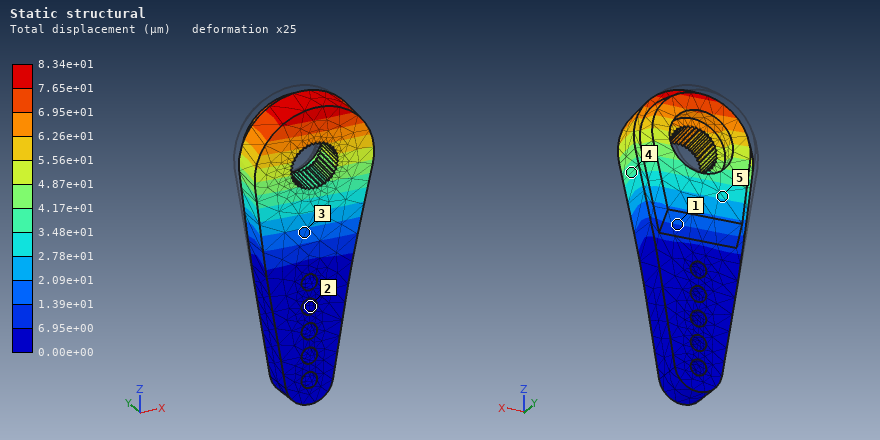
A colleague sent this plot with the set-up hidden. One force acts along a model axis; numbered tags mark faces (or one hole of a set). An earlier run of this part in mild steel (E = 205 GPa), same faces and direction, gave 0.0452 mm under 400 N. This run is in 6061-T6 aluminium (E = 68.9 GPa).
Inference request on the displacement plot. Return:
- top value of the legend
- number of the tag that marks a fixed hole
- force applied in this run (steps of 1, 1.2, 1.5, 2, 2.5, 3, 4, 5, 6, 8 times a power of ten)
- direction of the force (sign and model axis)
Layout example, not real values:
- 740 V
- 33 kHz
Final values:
- 8.34e+01 µm
- 2
- 250 N
- -Y
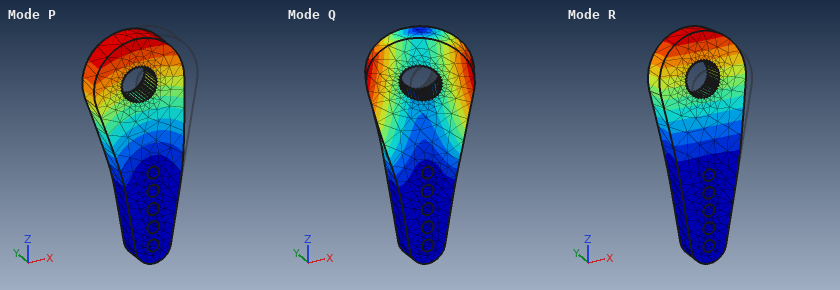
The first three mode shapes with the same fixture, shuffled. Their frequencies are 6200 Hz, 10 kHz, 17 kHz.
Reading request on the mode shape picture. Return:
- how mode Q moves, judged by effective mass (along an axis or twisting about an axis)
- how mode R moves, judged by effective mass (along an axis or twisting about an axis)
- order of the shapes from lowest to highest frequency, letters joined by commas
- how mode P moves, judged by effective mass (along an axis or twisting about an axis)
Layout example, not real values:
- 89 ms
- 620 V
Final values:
- twisting about Z
- along Y
- R, P, Q
- along X
